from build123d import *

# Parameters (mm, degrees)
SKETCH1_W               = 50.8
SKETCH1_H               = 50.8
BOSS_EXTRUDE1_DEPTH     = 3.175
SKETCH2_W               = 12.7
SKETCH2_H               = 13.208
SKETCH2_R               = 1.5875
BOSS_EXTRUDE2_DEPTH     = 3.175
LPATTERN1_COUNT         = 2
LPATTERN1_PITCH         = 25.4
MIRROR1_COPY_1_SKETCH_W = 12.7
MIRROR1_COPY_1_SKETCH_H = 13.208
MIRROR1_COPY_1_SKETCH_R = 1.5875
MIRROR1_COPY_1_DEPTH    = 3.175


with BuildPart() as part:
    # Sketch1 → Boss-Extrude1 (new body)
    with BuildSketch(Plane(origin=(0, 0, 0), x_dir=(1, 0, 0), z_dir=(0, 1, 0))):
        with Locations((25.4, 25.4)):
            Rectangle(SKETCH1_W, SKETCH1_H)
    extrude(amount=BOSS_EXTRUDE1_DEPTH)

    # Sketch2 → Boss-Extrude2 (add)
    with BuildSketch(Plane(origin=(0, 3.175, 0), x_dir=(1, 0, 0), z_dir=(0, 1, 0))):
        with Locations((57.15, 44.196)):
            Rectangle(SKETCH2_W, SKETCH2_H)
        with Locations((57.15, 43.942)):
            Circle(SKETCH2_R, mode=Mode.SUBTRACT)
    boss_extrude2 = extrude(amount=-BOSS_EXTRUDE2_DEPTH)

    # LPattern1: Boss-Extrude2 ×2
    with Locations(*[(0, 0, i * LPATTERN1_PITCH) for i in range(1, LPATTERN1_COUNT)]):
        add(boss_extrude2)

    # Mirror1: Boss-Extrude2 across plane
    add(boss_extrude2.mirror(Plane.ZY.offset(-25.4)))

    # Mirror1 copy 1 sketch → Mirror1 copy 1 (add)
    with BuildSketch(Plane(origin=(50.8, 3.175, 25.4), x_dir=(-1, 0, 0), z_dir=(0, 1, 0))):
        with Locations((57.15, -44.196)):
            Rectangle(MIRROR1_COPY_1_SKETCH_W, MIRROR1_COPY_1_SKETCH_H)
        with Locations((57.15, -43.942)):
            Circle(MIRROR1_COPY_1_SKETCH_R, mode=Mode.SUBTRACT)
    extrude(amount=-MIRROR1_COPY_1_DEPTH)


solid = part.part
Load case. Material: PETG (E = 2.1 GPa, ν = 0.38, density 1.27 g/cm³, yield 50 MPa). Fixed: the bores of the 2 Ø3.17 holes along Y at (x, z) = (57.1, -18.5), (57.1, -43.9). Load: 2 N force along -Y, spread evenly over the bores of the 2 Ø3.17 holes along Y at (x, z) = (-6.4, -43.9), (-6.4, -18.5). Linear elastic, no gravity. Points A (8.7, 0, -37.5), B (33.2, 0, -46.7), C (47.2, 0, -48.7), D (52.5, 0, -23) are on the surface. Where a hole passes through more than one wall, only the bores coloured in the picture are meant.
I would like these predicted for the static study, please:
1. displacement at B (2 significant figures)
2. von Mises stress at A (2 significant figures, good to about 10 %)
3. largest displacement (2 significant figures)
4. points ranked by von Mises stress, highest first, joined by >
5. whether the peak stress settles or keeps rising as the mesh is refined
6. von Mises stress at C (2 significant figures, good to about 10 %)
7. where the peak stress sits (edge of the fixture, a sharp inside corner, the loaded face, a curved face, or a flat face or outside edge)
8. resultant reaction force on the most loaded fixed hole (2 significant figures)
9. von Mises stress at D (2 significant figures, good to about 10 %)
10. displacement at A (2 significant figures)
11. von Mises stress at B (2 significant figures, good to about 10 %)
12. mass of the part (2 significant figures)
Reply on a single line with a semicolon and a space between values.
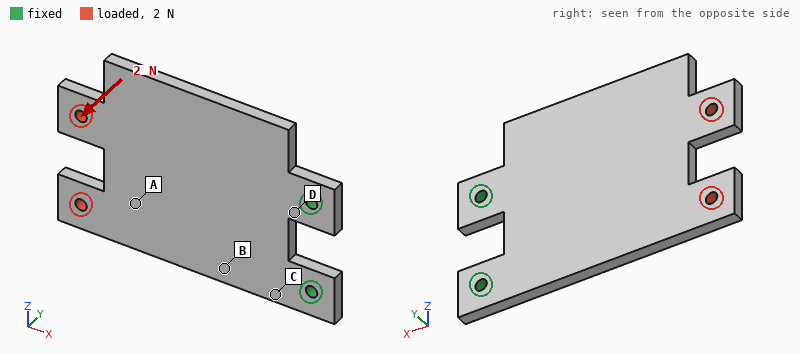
0.17 mm; 0.45 MPa; 0.93 mm; D > C > B > A; keeps rising; 1.9 MPa; edge of the fixture; 1.0 N; 2.5 MPa; 0.54 mm; 1.1 MPa; 13 g
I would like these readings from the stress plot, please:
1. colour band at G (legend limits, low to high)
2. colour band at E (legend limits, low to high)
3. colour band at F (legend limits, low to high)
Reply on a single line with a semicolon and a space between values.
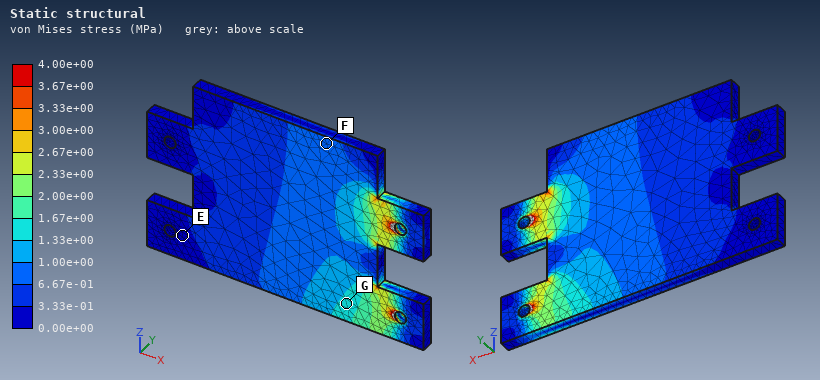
1.33e+00 to 1.67e+00 MPa; 0.00e+00 to 3.33e-01 MPa; 6.67e-01 to 1.00e+00 MPa
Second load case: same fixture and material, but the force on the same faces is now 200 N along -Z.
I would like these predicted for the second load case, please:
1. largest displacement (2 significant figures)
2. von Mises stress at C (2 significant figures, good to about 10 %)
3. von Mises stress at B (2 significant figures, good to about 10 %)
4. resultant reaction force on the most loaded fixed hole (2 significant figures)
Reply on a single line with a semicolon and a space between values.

0.95 mm; 8.5 MPa; 6.6 MPa; 470 N
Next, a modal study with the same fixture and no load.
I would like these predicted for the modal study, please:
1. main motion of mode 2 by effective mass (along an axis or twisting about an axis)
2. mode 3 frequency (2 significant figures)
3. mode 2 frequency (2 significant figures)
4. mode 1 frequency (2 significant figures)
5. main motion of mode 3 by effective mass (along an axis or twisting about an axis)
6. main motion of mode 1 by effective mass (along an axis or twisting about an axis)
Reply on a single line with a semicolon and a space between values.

twisting about X; 850 Hz; 400 Hz; 130 Hz; along Y; along Y
